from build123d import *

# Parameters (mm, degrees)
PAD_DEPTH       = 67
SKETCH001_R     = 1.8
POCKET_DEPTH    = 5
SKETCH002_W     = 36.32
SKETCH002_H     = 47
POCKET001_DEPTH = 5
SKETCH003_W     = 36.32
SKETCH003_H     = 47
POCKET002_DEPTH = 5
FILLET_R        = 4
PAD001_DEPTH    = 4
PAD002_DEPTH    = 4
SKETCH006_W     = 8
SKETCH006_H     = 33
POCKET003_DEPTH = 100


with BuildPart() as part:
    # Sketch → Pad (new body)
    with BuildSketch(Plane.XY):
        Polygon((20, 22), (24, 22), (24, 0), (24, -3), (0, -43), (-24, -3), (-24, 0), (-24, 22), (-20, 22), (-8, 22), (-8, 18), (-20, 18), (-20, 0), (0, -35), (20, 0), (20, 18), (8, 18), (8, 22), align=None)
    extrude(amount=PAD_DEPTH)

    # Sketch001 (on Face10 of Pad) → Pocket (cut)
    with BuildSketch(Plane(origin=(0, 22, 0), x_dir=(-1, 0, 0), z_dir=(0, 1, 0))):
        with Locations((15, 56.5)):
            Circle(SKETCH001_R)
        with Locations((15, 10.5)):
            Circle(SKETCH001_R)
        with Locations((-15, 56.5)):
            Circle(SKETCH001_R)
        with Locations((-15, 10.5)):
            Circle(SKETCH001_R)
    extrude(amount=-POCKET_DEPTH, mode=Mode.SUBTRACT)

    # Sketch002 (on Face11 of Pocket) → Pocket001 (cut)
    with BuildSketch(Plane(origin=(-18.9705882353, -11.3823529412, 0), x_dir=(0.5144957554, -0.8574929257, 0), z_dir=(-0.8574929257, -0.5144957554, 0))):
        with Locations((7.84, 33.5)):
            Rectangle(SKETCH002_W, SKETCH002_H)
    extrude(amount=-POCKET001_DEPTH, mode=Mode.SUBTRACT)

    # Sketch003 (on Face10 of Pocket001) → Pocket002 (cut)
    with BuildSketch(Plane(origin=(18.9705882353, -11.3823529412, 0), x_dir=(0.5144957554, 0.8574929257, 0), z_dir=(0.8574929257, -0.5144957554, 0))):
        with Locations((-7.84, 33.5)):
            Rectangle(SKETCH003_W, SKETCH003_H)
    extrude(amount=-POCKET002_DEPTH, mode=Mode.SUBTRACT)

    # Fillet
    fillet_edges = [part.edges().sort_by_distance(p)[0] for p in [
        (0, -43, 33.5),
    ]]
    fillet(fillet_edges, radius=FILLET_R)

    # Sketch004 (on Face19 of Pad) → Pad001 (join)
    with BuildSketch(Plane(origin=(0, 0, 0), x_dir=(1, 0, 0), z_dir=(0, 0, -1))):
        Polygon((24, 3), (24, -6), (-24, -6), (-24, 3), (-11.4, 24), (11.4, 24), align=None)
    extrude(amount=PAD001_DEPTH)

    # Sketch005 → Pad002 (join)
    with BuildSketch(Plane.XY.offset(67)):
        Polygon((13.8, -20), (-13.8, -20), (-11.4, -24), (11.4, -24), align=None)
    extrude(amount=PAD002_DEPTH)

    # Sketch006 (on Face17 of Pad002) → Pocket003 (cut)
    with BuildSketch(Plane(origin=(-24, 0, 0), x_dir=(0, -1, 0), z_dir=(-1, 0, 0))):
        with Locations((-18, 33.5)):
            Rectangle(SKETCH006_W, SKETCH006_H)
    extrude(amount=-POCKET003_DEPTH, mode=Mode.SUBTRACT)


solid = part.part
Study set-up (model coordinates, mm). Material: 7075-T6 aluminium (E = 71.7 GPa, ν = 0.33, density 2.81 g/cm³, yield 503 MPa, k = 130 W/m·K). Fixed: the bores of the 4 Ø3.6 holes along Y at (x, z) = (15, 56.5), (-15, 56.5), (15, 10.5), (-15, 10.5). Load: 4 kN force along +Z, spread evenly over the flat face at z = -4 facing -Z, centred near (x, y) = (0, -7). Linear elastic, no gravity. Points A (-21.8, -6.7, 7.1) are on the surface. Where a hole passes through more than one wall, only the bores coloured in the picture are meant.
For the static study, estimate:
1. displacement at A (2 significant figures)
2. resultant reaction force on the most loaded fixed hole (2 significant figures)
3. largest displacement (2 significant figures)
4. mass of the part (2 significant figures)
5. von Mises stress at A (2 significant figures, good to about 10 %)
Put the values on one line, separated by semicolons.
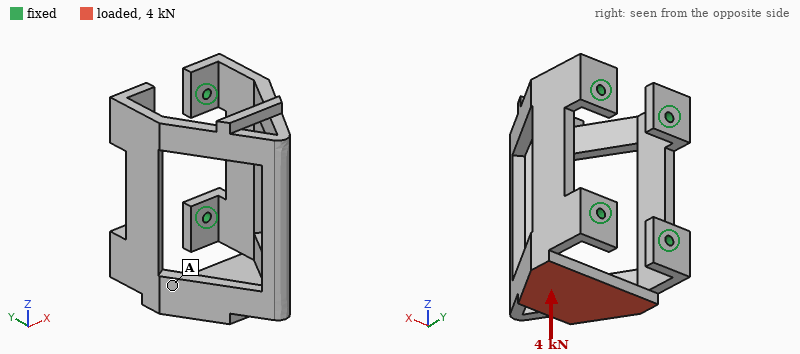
0.12 mm; 1.5 kN; 0.32 mm; 80 g; 37 MPa
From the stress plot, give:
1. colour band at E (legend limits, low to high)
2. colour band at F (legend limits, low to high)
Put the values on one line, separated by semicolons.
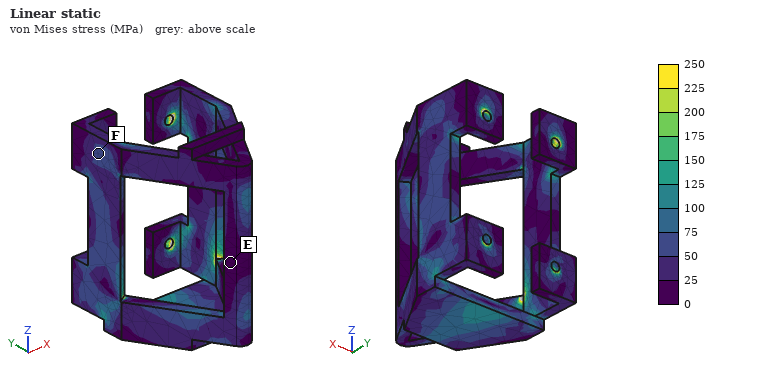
0 to 25 MPa; 50 to 75 MPa
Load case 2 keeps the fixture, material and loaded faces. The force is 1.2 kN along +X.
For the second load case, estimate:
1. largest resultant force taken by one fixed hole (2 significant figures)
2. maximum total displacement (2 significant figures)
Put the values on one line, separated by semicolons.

640 N; 0.20 mm
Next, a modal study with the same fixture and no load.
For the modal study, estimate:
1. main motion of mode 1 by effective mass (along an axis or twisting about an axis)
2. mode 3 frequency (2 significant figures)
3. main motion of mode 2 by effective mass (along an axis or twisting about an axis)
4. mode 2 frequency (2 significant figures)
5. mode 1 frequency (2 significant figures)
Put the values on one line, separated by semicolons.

along X; 2900 Hz; along Z; 2500 Hz; 1900 Hz
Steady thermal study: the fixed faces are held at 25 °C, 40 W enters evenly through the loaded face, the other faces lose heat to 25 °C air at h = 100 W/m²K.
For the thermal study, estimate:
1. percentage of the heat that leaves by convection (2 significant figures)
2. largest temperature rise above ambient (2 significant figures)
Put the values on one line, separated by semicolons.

54 %; 43 K
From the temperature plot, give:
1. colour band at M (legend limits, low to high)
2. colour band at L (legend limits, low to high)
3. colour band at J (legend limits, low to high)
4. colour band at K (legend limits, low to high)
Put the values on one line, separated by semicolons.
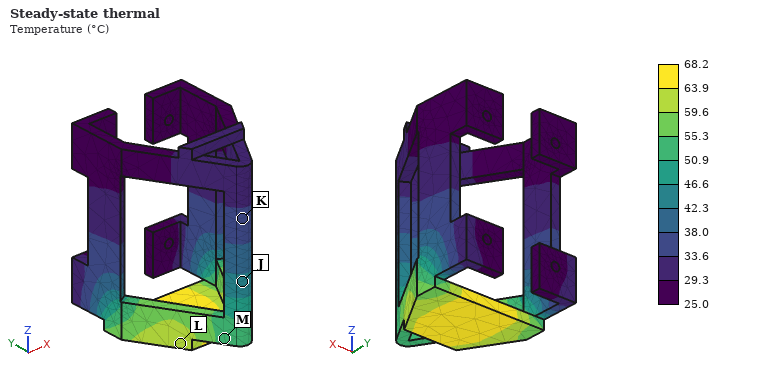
50.9 to 55.3 °C; 59.6 to 63.9 °C; 42.3 to 46.6 °C; 33.6 to 38.0 °C
